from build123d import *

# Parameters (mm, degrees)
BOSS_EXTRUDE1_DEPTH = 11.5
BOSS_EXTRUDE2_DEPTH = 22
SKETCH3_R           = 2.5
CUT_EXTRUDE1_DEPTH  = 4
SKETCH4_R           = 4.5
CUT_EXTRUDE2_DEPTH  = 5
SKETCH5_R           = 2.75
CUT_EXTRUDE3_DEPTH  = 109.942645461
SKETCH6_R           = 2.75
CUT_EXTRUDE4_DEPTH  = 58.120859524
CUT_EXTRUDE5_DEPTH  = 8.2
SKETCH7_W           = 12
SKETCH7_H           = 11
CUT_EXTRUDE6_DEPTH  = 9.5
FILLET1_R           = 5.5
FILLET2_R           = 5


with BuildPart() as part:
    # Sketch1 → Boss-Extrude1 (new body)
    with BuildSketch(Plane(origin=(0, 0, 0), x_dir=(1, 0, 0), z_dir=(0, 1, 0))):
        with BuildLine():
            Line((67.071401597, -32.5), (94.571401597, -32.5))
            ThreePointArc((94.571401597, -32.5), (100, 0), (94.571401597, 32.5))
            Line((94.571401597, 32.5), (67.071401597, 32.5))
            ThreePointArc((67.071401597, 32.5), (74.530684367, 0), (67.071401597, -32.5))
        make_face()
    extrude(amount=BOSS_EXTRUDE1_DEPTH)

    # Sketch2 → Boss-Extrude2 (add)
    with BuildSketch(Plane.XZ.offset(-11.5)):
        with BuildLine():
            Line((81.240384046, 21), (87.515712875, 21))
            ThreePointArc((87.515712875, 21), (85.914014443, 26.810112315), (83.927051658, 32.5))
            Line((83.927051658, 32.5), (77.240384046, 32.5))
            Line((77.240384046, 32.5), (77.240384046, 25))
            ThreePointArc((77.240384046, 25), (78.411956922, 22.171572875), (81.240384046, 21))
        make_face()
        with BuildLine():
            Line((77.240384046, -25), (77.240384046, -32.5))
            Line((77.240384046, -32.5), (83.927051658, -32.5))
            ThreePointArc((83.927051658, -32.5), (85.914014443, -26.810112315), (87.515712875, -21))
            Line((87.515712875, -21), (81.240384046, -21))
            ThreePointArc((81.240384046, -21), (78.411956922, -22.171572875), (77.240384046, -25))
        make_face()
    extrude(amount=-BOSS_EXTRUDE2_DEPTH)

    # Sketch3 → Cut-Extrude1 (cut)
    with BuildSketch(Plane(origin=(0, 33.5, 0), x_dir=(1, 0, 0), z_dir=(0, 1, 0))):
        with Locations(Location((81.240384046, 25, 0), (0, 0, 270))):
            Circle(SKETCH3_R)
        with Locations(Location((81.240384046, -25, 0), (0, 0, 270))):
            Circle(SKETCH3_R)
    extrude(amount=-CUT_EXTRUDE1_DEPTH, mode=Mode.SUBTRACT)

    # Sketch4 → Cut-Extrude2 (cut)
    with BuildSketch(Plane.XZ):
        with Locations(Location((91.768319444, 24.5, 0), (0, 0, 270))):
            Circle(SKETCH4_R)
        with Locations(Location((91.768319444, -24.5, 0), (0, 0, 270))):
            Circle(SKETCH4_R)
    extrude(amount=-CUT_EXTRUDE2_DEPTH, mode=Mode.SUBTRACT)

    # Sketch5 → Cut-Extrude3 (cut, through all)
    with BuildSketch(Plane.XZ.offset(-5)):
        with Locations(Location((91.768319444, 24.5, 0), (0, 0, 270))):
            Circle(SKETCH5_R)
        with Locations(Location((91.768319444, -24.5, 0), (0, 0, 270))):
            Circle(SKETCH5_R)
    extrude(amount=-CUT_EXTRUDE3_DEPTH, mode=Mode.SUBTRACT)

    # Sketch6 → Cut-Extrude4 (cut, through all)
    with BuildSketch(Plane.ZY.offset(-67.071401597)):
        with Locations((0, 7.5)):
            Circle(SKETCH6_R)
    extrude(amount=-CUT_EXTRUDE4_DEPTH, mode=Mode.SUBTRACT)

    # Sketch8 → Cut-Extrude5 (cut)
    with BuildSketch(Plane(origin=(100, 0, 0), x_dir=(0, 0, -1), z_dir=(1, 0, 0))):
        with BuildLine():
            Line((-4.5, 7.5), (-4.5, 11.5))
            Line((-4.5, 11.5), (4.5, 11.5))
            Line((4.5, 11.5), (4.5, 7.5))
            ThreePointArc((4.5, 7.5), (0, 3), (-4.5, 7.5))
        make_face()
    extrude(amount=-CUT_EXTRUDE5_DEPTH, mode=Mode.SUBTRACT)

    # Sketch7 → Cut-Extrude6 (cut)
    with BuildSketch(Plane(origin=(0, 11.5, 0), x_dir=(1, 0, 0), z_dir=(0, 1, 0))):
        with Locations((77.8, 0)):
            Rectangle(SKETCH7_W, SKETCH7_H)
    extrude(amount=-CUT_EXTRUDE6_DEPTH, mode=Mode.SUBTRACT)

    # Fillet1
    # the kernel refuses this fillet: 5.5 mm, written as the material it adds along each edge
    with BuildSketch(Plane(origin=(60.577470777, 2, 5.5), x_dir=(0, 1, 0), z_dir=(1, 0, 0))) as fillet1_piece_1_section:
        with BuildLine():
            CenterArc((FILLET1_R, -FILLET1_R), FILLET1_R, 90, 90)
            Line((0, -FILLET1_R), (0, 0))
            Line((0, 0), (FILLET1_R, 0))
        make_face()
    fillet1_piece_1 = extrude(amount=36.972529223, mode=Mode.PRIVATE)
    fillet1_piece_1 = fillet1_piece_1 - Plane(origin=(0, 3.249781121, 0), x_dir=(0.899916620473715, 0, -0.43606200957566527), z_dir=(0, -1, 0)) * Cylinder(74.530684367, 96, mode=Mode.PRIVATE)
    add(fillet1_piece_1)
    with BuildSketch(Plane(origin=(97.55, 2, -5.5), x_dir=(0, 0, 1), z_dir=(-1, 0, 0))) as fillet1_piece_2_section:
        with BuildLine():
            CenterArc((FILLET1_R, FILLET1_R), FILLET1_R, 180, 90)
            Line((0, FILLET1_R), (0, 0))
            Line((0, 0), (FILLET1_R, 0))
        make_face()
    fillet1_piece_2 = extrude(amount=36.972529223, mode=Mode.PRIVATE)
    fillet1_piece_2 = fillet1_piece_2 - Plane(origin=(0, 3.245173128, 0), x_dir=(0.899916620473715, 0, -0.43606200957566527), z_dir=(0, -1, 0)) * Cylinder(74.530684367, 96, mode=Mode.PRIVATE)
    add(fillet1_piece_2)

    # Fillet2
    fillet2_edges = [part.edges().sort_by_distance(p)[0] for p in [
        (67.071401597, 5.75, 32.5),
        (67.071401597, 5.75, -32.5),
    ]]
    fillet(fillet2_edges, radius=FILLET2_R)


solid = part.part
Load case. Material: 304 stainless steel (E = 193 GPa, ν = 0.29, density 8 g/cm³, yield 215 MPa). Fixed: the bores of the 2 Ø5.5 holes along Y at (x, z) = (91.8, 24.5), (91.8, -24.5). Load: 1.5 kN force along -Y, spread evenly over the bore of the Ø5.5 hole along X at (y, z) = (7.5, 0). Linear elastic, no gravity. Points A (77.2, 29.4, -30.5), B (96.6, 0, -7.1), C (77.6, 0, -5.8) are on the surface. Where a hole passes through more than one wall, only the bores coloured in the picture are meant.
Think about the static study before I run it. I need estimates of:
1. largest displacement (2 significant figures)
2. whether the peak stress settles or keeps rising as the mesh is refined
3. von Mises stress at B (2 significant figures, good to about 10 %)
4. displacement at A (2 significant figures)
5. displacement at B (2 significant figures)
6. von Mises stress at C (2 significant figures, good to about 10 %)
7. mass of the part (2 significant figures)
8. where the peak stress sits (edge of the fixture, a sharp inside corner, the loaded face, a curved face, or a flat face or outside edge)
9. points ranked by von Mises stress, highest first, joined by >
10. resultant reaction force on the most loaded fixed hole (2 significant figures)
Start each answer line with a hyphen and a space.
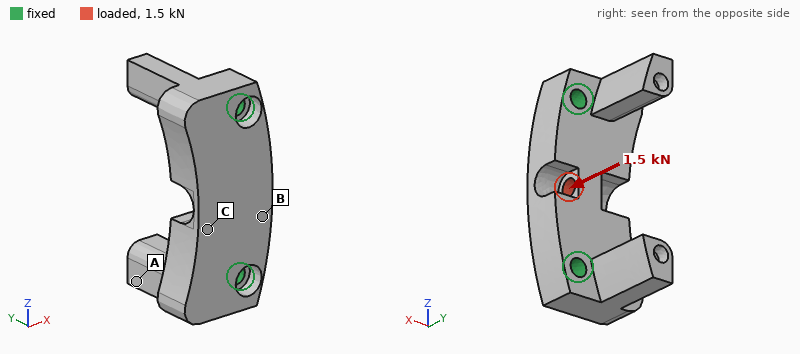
- 6.5 µm
- keeps rising
- 19 MPa
- 4.9 µm
- 3.4 µm
- 14 MPa
- 170 g
- edge of the fixture
- B > C > A
- 1.1 kN
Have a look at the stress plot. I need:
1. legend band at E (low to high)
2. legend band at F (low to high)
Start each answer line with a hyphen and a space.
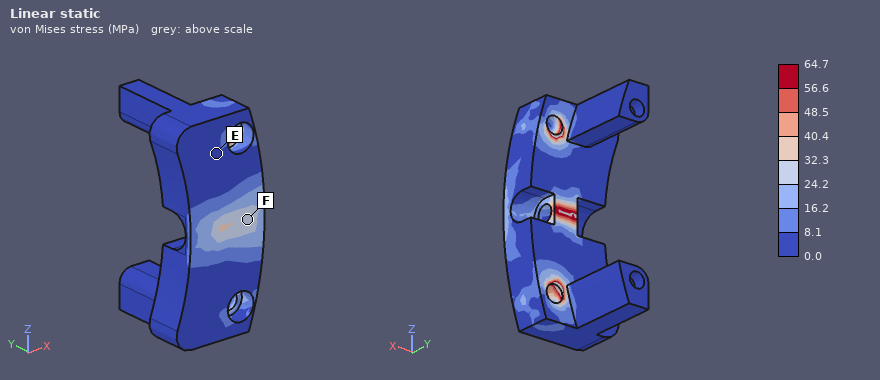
- 0.0 to 8.1 MPa
- 24.2 to 32.3 MPa
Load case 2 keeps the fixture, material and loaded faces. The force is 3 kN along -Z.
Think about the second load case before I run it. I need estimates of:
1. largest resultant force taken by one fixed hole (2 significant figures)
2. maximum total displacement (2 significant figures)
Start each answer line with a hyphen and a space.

- 1.5 kN
- 2.2 µm
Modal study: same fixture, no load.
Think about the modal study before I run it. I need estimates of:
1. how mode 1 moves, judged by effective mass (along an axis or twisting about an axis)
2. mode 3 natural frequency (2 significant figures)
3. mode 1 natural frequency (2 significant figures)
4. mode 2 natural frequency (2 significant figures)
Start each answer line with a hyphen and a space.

- along Y
- 9000 Hz
- 6400 Hz
- 7700 Hz
